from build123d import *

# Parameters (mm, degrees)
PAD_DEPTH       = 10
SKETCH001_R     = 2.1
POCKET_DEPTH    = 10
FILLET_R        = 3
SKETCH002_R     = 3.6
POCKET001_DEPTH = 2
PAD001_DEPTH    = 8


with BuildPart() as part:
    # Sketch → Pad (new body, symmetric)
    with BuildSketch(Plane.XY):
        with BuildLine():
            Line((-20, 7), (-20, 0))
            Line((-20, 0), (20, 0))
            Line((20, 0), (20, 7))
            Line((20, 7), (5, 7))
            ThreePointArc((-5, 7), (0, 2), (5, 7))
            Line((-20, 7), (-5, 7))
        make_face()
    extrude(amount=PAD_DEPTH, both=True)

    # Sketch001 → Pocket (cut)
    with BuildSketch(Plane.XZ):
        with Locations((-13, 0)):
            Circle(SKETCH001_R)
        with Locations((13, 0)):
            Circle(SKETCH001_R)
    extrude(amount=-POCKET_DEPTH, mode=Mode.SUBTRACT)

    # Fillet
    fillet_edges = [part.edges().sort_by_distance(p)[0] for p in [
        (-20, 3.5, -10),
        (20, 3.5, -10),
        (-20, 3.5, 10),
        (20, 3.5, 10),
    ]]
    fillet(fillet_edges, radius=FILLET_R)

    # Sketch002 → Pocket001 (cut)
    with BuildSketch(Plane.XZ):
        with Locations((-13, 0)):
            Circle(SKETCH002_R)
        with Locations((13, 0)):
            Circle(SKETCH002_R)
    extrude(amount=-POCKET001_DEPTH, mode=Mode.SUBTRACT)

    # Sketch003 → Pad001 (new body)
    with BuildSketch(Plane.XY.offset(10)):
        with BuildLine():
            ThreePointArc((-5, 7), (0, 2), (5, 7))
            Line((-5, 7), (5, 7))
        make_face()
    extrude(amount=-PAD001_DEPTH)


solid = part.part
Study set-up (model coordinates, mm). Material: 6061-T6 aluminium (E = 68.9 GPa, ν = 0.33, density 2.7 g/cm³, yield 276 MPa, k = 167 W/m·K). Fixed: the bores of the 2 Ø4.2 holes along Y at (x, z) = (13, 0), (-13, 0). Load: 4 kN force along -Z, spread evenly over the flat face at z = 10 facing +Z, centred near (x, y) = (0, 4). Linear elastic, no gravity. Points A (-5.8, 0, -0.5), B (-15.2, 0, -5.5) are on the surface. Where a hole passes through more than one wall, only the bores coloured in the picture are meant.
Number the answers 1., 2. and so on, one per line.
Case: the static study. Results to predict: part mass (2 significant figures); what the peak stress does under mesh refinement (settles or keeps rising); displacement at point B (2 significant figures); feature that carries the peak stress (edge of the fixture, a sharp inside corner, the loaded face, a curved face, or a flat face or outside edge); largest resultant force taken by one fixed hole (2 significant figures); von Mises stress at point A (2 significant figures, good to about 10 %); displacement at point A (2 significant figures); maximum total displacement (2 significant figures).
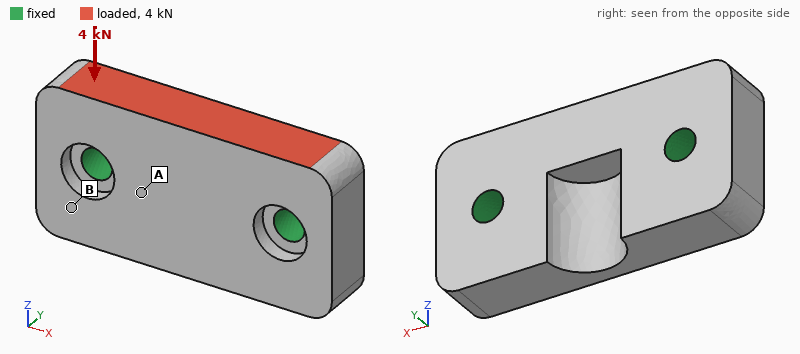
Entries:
1. 13 g
2. keeps rising
3. 2.1 µm
4. edge of the fixture
5. 2.1 kN
6. 19 MPa
7. 5.9 µm
8. 9.8 µm
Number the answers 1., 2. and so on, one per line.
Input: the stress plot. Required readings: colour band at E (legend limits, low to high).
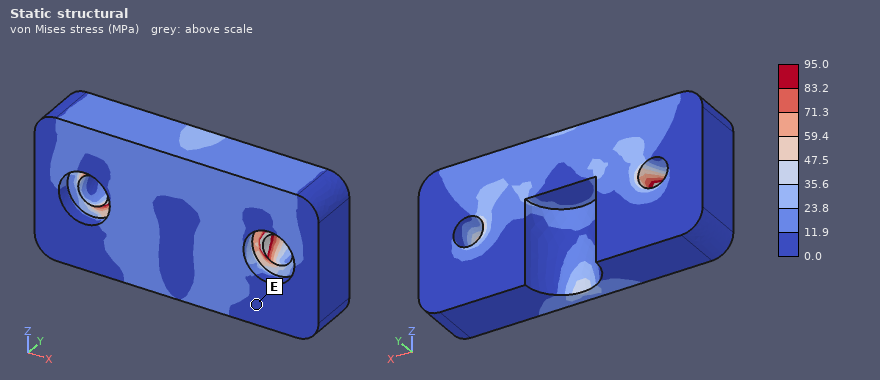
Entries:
1. 0.0 to 11.9 MPa
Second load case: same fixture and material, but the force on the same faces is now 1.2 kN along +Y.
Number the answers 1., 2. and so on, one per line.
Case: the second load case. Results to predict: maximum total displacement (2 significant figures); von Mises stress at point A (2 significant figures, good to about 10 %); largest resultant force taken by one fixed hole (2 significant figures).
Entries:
1. 22 µm
2. 23 MPa
3. 610 N
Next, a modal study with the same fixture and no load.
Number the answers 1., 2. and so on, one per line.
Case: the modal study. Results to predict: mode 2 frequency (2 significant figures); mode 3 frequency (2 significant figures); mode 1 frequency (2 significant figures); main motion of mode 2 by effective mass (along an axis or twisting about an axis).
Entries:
1. 31 kHz
2. 34 kHz
3. 24 kHz
4. along Y
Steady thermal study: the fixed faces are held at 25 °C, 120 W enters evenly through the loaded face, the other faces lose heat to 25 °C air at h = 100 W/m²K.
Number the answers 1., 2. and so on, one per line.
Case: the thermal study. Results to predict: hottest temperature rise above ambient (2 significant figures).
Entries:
1. 43 K
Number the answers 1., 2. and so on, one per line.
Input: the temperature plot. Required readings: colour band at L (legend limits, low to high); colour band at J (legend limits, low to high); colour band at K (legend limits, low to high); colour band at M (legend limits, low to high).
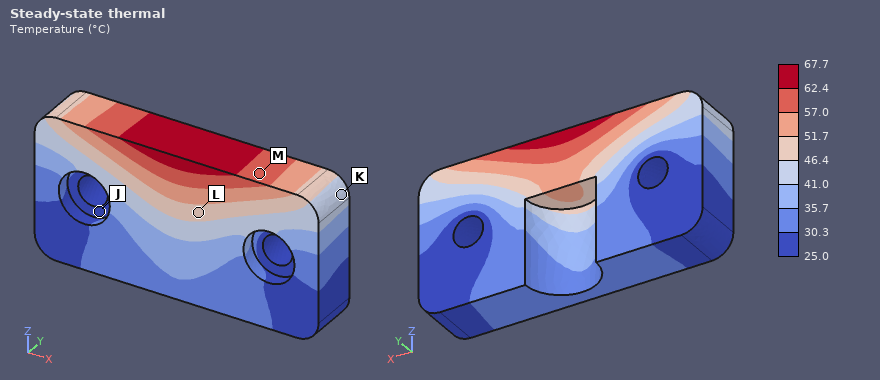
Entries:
1. 46.4 to 51.7 °C
2. 25.0 to 30.3 °C
3. 41.0 to 46.4 °C
4. 57.0 to 62.4 °C
